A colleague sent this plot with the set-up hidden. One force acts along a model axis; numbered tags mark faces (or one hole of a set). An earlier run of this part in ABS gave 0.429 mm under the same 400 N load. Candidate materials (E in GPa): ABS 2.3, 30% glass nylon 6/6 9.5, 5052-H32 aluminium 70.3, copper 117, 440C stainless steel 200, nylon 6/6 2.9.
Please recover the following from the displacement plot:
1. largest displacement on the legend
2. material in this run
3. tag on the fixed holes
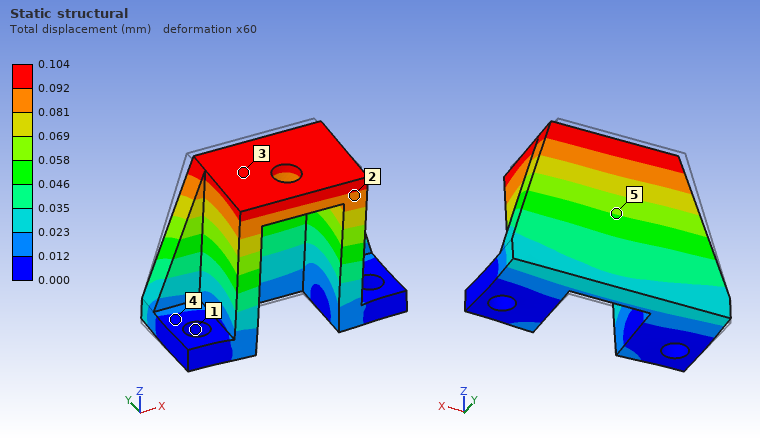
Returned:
0.104 mm
30% glass nylon 6/6
1
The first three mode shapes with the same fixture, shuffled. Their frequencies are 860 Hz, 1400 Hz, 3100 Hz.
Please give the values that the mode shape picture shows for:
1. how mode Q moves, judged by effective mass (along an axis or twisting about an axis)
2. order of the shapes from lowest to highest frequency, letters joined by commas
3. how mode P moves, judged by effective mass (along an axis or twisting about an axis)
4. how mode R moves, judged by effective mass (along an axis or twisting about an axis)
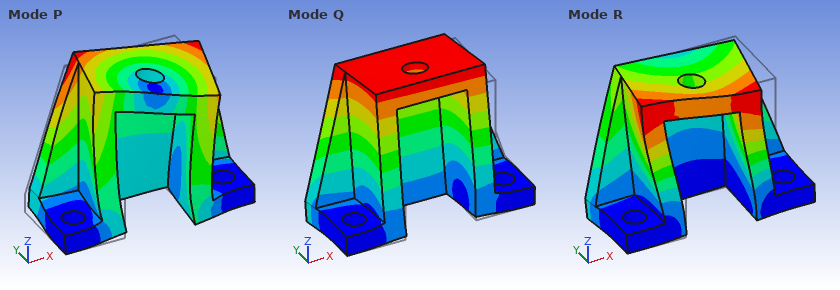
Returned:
along Y
Q, R, P
along X
along X
